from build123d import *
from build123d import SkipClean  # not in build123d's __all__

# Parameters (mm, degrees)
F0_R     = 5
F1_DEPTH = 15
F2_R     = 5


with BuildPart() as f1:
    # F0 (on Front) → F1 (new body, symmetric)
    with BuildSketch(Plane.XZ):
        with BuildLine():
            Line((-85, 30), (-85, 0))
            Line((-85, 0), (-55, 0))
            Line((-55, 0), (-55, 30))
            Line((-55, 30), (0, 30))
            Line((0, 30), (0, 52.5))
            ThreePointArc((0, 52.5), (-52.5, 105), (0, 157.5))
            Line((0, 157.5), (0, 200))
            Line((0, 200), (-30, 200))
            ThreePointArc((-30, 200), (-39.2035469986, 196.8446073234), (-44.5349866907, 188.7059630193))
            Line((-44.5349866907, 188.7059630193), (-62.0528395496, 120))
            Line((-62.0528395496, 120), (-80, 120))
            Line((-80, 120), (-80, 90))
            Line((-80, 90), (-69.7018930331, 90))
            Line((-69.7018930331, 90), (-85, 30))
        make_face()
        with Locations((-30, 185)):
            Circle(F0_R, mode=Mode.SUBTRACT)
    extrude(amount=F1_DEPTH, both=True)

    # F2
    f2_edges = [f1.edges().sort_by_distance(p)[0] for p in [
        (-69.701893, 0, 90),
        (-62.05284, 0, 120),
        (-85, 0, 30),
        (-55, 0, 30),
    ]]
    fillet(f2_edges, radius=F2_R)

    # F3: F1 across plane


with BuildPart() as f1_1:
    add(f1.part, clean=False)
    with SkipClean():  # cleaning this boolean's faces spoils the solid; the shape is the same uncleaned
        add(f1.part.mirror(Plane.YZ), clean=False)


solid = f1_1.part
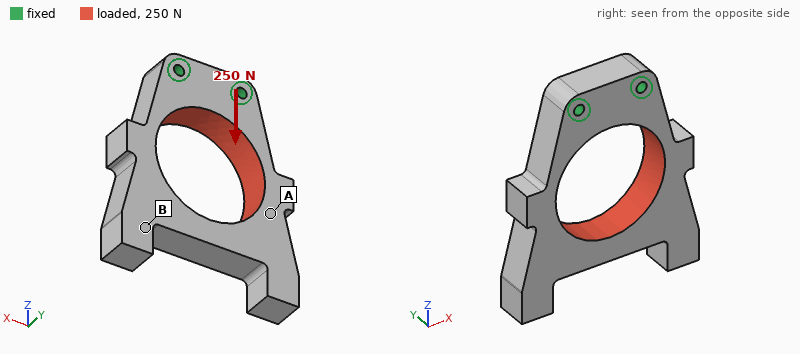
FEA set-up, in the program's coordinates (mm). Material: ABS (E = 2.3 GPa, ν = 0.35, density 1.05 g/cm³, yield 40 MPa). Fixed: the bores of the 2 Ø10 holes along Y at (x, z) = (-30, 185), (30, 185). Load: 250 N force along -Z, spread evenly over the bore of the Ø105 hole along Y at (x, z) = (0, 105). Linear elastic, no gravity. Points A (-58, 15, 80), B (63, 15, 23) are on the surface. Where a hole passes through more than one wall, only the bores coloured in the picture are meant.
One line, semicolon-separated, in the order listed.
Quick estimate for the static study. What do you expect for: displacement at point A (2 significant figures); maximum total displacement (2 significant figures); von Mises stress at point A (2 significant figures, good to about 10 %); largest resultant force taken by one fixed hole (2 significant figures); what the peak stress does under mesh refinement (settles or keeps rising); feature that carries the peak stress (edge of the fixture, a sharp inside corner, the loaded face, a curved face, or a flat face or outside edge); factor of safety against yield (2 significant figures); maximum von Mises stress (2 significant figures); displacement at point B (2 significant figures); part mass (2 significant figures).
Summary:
21 µm; 34 µm; 0.11 MPa; 130 N; settles; the loaded face; 62; 0.65 MPa; 17 µm; 480 g
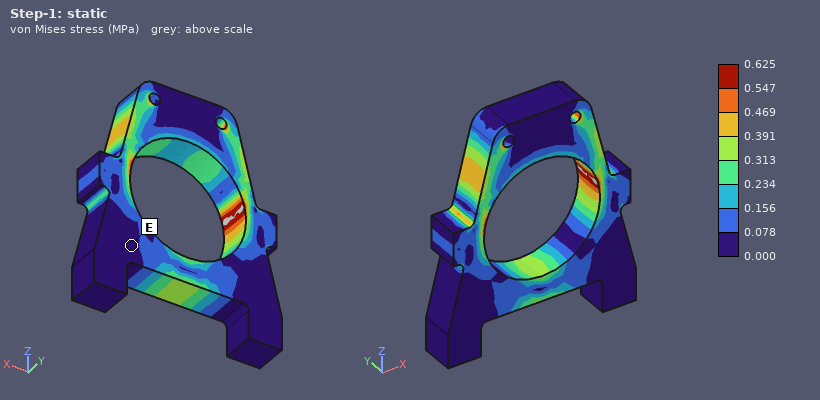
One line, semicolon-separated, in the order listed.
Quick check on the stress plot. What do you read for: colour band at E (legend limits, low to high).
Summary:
0.000 to 0.078 MPa
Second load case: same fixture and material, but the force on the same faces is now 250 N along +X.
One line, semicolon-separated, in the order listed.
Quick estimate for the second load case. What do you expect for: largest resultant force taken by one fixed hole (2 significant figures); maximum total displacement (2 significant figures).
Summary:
310 N; 0.30 mm
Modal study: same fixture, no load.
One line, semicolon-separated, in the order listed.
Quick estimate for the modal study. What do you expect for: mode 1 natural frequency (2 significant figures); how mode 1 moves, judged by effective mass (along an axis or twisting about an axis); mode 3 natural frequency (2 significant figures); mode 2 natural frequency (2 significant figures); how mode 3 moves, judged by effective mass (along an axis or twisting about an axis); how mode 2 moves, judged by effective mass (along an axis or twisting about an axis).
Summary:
130 Hz; along Y; 260 Hz; 210 Hz; twisting about Z; along X
